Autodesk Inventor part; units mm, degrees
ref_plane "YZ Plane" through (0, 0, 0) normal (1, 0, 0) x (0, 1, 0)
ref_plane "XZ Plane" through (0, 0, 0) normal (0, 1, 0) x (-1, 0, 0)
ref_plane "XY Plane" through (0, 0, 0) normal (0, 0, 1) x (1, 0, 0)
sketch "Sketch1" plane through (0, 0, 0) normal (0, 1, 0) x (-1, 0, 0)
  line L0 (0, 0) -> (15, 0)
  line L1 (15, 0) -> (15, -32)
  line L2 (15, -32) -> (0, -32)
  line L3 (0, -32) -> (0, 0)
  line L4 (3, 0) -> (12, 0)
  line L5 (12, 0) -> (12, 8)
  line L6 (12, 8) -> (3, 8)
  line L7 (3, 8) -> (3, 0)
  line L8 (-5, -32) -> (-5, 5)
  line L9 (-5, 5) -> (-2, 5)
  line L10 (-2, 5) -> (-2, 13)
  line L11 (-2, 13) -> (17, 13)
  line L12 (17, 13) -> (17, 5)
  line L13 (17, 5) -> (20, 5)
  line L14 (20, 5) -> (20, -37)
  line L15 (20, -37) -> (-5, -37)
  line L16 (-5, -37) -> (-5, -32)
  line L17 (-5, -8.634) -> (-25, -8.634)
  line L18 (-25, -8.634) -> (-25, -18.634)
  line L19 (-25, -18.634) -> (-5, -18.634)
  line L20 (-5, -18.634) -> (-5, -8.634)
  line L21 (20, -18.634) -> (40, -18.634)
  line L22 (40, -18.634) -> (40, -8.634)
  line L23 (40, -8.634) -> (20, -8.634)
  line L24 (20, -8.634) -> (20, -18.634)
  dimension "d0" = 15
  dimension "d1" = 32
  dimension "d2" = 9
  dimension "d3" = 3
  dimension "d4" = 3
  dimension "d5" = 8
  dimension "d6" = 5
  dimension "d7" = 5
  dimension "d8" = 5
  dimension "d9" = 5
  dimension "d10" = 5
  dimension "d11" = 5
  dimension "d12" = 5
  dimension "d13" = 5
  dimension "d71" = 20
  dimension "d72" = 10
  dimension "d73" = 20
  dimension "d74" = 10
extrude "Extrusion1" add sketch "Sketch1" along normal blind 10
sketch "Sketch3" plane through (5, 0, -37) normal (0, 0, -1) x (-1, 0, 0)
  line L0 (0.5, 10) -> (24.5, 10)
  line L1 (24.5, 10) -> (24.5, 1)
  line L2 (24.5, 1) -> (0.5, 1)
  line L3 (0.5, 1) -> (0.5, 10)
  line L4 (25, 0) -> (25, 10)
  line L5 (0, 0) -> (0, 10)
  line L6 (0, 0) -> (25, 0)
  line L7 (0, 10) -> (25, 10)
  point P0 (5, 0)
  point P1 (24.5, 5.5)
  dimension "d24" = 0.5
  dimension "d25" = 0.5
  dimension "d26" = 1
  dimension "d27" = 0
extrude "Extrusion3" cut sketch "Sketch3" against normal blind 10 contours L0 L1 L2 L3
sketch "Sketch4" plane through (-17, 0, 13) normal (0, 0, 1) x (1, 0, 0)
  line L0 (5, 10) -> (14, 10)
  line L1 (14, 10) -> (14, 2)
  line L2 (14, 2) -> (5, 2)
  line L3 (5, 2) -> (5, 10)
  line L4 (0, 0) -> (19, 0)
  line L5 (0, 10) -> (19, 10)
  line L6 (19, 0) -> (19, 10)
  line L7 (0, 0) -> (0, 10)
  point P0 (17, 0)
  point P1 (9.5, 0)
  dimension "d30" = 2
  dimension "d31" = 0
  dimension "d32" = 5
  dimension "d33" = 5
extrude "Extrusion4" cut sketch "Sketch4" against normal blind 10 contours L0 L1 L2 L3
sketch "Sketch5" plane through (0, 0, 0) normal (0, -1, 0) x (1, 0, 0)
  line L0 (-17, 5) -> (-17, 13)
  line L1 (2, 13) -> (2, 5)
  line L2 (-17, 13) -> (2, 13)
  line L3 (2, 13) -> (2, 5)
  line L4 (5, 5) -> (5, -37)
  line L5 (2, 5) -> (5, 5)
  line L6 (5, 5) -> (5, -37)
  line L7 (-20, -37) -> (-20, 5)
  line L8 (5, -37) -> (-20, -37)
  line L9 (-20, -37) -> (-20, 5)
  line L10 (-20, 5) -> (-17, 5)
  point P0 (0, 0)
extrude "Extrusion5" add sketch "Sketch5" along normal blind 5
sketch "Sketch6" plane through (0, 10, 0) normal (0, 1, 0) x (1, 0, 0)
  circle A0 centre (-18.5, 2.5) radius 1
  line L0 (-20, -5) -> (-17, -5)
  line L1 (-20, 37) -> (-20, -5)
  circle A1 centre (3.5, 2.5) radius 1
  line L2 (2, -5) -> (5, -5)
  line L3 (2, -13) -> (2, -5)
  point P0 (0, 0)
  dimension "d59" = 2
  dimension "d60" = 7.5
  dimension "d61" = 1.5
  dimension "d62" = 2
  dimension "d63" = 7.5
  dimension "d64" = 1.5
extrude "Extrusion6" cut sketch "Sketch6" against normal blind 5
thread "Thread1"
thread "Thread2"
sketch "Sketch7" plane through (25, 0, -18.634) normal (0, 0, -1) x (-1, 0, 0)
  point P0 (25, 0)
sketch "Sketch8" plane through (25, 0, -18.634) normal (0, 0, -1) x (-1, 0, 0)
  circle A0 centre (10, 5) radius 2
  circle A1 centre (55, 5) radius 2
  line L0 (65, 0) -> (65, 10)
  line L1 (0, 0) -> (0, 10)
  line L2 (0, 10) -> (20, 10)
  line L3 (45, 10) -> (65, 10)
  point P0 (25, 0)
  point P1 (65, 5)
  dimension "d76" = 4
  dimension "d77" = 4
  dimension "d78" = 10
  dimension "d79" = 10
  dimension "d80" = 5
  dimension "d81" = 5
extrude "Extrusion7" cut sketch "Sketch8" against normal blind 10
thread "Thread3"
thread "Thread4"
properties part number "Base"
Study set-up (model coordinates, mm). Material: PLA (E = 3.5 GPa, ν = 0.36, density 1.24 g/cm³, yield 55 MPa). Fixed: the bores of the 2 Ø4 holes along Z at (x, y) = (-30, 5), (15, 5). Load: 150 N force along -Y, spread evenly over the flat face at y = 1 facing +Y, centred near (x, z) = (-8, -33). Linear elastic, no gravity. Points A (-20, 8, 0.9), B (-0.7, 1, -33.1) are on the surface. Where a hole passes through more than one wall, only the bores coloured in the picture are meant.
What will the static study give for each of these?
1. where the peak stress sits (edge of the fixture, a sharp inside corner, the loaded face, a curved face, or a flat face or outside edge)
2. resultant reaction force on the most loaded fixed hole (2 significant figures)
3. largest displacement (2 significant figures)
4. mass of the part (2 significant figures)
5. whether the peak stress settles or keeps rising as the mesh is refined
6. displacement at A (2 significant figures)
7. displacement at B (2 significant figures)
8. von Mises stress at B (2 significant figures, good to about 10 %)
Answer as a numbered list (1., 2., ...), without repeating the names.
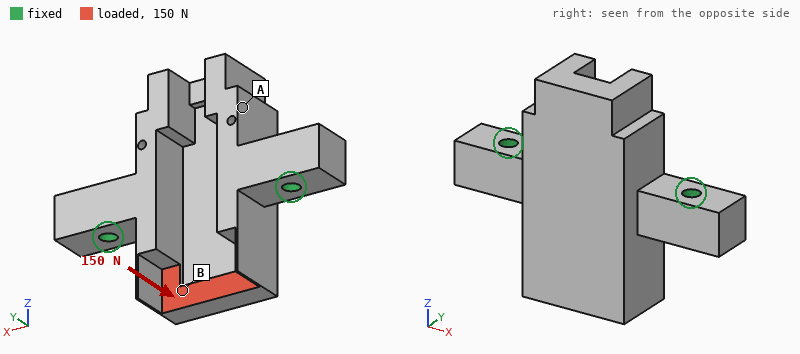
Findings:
1. edge of the fixture
2. 99 N
3. 0.33 mm
4. 18 g
5. keeps rising
6. 0.11 mm
7. 0.24 mm
8. 2.6 MPa
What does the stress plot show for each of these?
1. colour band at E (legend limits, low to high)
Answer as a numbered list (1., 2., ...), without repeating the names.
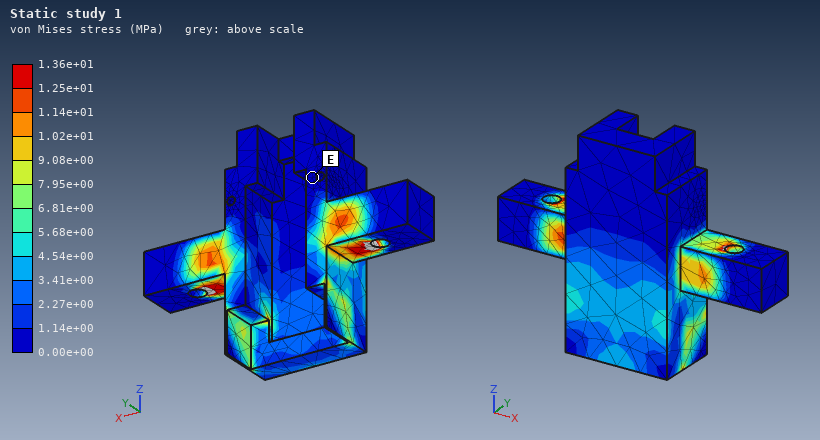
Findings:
1. 0.00e+00 to 1.14e+00 MPa
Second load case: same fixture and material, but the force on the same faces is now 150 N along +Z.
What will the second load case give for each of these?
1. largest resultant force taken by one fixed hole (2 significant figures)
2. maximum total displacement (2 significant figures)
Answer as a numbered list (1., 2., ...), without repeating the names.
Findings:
1. 75 N
2. 60 µm
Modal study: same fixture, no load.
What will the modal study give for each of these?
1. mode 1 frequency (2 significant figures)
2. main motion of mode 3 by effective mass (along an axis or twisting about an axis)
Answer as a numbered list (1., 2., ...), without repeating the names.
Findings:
1. 1600 Hz
2. along Y
